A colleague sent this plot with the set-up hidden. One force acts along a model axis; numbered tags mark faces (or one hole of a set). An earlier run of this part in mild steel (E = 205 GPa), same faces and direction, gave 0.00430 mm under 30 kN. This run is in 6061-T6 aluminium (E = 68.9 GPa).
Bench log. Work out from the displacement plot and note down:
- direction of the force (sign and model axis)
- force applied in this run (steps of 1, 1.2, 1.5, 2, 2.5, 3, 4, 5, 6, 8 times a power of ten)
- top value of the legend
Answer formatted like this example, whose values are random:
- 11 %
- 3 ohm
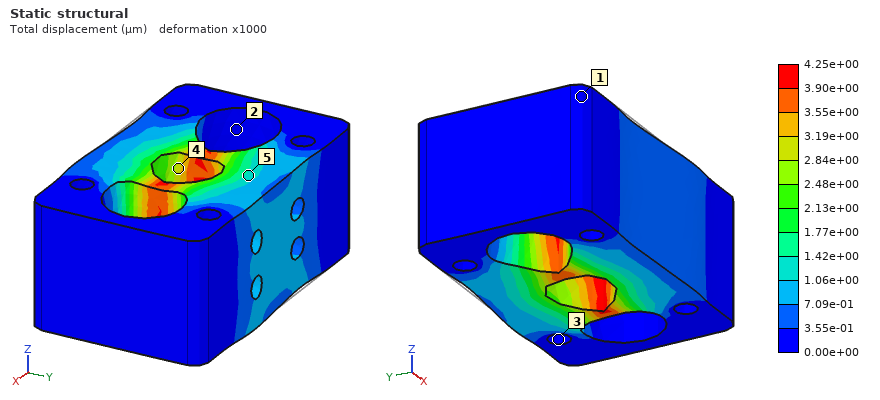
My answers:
- +X
- 10 kN
- 4.25e+00 µm
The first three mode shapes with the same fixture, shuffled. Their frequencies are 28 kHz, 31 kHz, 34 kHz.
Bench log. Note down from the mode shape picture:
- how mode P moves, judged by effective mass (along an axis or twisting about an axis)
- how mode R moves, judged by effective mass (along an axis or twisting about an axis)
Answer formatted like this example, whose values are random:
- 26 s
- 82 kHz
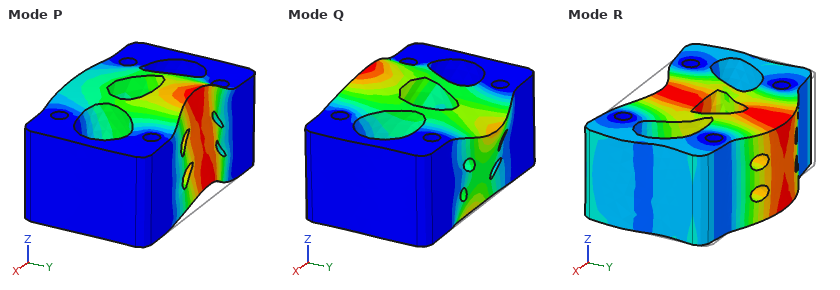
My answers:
- along Z
- along Y
